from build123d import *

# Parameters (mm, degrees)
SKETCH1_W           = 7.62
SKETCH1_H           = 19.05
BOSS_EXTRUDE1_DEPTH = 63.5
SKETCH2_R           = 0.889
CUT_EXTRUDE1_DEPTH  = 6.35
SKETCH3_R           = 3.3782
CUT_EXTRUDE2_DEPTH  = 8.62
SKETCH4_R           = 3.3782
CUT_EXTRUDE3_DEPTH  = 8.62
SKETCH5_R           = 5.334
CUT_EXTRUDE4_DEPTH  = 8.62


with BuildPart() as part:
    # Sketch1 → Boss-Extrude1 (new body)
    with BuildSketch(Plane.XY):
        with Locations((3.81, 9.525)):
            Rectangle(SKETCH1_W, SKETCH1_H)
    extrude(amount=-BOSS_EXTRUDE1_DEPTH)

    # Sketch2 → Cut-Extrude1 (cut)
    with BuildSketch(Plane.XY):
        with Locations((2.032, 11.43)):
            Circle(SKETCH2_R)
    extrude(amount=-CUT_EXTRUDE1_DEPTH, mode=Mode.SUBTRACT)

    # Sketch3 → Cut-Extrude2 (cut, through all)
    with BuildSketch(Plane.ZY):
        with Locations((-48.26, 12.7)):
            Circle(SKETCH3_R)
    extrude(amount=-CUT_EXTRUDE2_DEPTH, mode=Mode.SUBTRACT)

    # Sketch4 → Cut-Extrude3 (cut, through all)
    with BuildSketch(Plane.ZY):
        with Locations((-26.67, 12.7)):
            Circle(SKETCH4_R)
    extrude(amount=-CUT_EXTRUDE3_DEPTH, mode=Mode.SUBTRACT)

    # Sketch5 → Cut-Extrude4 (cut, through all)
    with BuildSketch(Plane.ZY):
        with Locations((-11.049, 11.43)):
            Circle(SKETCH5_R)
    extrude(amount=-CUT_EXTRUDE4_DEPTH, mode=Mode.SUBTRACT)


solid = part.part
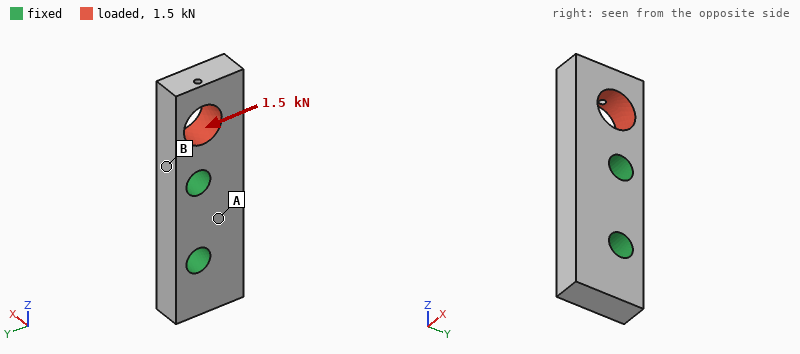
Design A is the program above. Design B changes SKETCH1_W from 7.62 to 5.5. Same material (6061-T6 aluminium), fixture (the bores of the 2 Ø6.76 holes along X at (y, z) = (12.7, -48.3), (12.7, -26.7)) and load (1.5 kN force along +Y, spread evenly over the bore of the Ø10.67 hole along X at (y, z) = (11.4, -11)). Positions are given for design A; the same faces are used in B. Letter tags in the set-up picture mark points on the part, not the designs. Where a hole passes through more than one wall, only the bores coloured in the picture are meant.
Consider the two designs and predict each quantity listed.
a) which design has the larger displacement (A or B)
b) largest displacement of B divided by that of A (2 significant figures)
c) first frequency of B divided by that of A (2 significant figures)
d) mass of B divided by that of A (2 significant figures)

B
1.4
0.77
0.72
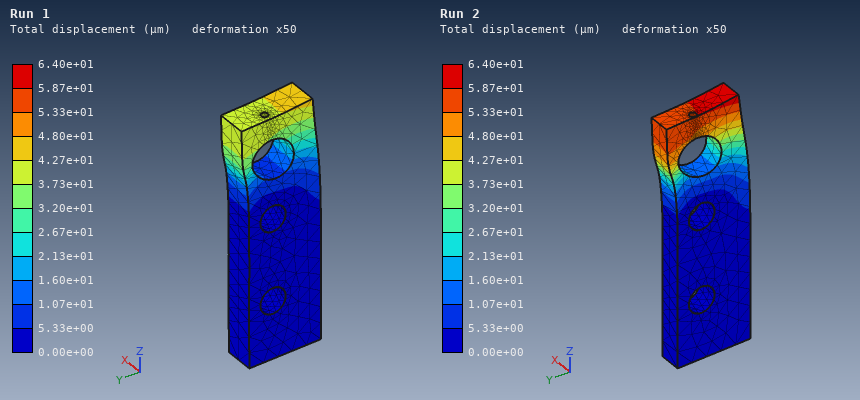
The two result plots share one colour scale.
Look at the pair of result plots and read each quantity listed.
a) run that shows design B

Run 2
